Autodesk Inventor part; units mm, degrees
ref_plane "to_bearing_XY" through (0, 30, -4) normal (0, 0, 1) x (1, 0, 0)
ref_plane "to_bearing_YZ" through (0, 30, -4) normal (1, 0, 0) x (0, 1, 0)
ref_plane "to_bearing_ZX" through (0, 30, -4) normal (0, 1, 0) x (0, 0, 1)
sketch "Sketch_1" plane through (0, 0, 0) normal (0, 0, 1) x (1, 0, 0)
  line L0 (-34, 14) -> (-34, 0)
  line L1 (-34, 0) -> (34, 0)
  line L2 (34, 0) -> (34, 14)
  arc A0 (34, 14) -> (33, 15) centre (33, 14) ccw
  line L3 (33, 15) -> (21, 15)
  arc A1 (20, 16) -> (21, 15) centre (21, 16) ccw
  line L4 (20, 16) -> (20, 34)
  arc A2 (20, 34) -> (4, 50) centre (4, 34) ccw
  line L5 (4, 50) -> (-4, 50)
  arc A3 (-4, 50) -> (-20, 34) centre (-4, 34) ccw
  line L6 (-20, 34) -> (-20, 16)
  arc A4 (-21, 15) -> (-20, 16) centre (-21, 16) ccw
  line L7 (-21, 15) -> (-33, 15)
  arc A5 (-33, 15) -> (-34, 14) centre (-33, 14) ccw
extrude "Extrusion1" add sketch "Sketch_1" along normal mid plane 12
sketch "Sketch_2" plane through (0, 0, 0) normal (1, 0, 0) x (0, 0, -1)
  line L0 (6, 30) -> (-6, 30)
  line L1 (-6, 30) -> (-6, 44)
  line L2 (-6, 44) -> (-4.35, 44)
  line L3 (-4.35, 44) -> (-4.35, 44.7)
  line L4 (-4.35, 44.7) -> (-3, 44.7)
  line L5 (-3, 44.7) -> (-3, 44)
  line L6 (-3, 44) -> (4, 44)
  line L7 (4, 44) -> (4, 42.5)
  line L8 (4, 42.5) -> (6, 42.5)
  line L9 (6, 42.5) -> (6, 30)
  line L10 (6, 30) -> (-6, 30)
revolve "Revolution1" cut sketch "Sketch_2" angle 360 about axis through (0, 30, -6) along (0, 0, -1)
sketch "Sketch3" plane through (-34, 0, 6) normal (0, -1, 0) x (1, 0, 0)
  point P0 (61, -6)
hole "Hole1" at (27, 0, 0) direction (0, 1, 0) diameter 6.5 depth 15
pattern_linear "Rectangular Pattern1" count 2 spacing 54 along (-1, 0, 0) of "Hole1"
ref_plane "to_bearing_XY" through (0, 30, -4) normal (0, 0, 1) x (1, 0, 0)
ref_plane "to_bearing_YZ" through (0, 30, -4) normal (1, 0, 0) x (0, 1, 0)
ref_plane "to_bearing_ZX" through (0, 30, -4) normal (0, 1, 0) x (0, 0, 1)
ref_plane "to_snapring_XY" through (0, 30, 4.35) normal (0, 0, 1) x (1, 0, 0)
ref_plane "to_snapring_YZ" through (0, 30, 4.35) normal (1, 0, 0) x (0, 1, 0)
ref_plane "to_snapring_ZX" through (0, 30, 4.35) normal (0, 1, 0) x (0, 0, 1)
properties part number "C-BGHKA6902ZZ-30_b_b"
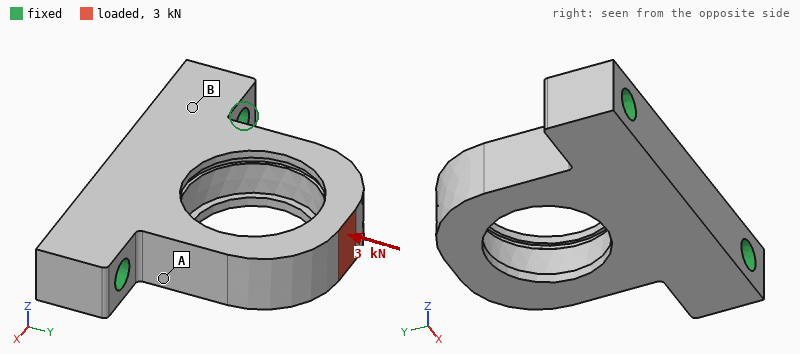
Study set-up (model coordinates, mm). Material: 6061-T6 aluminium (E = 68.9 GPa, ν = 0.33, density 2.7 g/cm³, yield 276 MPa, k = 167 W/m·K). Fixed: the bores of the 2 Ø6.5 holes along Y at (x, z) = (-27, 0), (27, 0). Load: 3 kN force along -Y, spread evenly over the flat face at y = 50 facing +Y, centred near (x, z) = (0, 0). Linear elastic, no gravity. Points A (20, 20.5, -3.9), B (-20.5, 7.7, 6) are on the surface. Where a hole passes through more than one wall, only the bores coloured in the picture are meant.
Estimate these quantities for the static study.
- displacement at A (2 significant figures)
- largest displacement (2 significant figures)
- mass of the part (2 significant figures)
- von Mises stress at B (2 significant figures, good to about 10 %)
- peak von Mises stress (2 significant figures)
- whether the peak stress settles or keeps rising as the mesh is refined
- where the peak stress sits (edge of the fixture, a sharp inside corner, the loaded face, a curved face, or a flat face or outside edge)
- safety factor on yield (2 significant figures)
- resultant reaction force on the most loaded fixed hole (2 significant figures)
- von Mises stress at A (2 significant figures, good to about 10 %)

8.6 µm
51 µm
53 g
14 MPa
150 MPa
settles
a curved face
1.8
1.6 kN
40 MPa
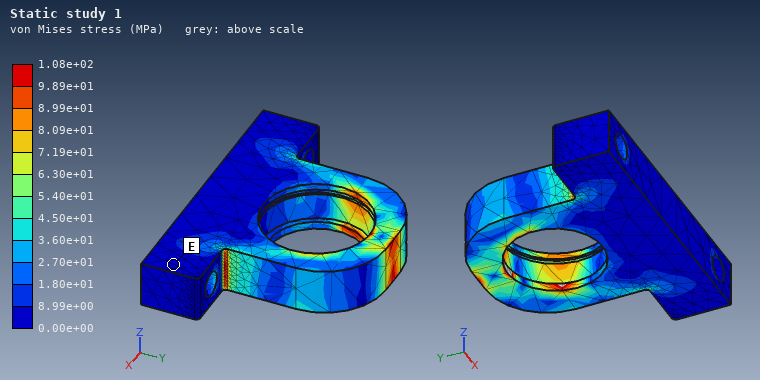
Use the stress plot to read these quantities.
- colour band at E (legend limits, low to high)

0.00e+00 to 8.99e+00 MPa
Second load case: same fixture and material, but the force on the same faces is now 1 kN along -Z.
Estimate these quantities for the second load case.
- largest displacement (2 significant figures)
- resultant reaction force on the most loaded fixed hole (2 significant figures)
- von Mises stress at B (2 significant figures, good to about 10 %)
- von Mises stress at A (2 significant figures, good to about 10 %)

0.21 mm
500 N
60 MPa
51 MPa
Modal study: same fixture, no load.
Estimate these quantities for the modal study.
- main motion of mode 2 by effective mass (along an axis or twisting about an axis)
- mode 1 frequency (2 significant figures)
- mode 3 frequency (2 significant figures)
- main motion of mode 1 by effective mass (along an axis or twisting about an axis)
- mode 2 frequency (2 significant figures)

along X
4200 Hz
10 kHz
along Z
7800 Hz
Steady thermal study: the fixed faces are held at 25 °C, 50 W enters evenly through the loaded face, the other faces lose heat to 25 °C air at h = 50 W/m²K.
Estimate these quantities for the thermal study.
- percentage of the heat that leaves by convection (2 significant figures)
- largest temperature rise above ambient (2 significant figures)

14 %
77 K
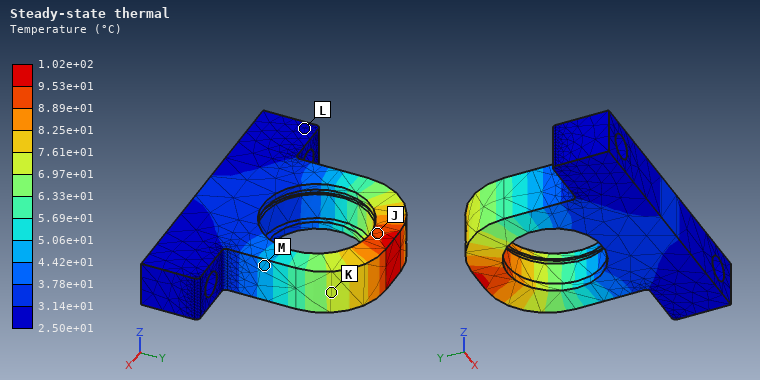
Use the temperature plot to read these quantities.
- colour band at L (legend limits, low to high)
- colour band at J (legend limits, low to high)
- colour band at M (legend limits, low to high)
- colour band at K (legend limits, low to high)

2.50e+01 to 3.14e+01 °C
8.89e+01 to 9.53e+01 °C
4.42e+01 to 5.06e+01 °C
6.97e+01 to 7.61e+01 °C
